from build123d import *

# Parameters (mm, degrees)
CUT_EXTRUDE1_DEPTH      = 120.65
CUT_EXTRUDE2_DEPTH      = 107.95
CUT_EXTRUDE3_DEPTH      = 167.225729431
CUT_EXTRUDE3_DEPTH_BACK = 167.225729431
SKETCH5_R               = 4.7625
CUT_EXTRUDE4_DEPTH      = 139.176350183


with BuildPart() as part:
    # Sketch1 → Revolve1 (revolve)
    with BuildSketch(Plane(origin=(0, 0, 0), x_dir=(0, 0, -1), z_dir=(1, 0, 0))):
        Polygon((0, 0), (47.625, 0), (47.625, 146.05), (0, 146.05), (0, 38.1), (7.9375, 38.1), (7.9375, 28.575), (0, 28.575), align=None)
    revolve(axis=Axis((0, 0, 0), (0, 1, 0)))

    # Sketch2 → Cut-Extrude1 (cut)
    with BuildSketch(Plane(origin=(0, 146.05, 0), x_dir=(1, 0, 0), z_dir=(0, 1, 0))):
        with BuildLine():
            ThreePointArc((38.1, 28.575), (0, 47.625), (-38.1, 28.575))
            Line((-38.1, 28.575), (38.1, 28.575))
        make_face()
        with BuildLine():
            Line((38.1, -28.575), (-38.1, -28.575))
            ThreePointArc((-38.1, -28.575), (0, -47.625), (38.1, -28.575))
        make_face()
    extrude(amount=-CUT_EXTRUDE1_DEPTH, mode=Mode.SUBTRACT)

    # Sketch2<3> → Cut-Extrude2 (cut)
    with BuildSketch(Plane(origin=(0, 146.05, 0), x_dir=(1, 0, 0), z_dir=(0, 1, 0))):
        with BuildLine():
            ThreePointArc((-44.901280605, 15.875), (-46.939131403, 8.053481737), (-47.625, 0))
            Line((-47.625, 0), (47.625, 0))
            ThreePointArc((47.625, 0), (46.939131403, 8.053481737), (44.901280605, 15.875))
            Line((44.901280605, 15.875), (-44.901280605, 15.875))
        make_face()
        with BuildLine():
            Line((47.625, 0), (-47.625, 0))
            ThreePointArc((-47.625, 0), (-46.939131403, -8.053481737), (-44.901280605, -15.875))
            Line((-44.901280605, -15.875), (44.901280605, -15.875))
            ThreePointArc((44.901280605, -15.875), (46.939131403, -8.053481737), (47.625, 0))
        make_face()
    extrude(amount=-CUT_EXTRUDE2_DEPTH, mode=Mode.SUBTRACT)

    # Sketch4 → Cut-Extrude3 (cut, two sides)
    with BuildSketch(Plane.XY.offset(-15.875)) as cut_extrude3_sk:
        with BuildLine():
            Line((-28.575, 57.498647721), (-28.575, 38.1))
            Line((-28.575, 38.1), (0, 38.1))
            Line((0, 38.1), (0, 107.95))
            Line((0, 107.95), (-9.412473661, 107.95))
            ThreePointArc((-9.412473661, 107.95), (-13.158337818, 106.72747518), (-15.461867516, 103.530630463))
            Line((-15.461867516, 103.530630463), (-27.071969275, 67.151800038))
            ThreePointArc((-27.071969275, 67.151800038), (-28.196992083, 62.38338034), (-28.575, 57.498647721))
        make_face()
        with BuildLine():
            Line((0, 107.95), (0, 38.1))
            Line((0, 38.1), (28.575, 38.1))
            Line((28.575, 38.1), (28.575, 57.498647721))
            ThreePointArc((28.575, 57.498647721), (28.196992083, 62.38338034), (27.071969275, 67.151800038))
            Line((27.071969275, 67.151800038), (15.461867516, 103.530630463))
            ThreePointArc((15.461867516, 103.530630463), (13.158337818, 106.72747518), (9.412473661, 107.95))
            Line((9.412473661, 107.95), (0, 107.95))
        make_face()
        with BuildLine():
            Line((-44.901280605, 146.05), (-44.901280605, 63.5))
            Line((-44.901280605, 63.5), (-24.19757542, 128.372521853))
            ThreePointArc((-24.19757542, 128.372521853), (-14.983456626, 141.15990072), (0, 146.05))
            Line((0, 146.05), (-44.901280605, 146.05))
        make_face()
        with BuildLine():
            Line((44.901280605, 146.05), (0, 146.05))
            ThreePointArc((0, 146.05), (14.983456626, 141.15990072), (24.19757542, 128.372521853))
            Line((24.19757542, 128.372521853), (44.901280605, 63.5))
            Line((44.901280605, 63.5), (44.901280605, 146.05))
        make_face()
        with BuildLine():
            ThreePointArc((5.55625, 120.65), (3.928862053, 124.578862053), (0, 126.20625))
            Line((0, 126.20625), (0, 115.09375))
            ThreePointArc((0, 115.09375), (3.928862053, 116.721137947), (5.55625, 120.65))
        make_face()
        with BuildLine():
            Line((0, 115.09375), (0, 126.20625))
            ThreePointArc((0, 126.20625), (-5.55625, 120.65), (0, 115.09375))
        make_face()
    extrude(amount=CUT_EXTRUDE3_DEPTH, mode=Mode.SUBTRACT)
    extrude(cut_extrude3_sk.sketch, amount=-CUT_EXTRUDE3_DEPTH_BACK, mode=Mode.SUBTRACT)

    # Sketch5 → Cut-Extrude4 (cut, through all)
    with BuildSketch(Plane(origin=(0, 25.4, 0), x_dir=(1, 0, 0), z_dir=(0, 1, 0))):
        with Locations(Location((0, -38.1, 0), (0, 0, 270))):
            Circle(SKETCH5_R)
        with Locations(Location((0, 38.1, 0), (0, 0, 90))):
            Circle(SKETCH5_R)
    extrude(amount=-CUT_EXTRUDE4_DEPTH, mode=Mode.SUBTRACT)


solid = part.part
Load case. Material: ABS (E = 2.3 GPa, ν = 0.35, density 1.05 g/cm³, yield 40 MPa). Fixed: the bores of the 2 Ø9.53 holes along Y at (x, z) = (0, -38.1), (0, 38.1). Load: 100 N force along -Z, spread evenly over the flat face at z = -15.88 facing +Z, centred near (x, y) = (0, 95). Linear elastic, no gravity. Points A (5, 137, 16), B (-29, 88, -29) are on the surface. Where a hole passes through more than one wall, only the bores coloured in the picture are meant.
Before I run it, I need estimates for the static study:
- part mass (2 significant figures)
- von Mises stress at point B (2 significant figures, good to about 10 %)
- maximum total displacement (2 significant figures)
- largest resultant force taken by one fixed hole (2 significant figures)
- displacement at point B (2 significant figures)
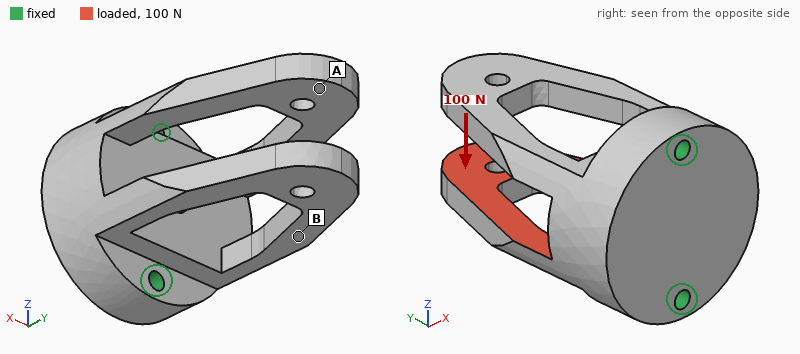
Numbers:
350 g
2.0 MPa
2.0 mm
130 N
0.72 mm
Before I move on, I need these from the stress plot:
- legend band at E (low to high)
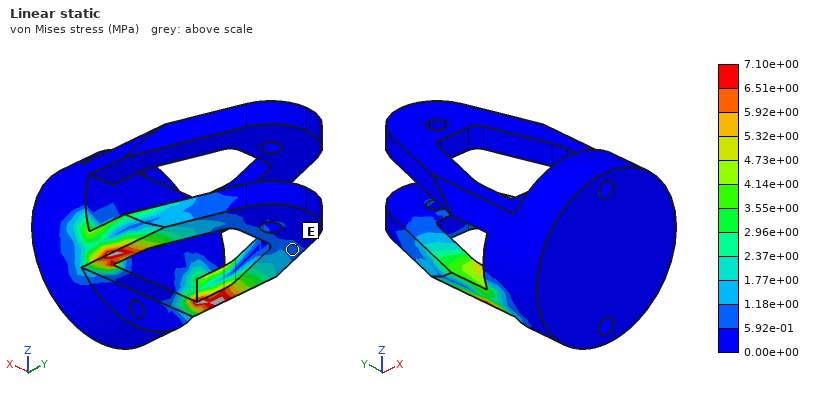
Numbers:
5.92e-01 to 1.18e+00 MPa
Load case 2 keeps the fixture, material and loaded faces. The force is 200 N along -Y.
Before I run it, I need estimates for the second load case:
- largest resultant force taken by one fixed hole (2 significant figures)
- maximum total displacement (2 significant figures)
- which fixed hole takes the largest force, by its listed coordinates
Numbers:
150 N
0.51 mm
(0, -38.1)
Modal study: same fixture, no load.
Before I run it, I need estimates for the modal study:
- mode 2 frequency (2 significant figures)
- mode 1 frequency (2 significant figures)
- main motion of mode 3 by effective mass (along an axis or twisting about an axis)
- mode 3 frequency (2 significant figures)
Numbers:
190 Hz
190 Hz
along X
450 Hz
